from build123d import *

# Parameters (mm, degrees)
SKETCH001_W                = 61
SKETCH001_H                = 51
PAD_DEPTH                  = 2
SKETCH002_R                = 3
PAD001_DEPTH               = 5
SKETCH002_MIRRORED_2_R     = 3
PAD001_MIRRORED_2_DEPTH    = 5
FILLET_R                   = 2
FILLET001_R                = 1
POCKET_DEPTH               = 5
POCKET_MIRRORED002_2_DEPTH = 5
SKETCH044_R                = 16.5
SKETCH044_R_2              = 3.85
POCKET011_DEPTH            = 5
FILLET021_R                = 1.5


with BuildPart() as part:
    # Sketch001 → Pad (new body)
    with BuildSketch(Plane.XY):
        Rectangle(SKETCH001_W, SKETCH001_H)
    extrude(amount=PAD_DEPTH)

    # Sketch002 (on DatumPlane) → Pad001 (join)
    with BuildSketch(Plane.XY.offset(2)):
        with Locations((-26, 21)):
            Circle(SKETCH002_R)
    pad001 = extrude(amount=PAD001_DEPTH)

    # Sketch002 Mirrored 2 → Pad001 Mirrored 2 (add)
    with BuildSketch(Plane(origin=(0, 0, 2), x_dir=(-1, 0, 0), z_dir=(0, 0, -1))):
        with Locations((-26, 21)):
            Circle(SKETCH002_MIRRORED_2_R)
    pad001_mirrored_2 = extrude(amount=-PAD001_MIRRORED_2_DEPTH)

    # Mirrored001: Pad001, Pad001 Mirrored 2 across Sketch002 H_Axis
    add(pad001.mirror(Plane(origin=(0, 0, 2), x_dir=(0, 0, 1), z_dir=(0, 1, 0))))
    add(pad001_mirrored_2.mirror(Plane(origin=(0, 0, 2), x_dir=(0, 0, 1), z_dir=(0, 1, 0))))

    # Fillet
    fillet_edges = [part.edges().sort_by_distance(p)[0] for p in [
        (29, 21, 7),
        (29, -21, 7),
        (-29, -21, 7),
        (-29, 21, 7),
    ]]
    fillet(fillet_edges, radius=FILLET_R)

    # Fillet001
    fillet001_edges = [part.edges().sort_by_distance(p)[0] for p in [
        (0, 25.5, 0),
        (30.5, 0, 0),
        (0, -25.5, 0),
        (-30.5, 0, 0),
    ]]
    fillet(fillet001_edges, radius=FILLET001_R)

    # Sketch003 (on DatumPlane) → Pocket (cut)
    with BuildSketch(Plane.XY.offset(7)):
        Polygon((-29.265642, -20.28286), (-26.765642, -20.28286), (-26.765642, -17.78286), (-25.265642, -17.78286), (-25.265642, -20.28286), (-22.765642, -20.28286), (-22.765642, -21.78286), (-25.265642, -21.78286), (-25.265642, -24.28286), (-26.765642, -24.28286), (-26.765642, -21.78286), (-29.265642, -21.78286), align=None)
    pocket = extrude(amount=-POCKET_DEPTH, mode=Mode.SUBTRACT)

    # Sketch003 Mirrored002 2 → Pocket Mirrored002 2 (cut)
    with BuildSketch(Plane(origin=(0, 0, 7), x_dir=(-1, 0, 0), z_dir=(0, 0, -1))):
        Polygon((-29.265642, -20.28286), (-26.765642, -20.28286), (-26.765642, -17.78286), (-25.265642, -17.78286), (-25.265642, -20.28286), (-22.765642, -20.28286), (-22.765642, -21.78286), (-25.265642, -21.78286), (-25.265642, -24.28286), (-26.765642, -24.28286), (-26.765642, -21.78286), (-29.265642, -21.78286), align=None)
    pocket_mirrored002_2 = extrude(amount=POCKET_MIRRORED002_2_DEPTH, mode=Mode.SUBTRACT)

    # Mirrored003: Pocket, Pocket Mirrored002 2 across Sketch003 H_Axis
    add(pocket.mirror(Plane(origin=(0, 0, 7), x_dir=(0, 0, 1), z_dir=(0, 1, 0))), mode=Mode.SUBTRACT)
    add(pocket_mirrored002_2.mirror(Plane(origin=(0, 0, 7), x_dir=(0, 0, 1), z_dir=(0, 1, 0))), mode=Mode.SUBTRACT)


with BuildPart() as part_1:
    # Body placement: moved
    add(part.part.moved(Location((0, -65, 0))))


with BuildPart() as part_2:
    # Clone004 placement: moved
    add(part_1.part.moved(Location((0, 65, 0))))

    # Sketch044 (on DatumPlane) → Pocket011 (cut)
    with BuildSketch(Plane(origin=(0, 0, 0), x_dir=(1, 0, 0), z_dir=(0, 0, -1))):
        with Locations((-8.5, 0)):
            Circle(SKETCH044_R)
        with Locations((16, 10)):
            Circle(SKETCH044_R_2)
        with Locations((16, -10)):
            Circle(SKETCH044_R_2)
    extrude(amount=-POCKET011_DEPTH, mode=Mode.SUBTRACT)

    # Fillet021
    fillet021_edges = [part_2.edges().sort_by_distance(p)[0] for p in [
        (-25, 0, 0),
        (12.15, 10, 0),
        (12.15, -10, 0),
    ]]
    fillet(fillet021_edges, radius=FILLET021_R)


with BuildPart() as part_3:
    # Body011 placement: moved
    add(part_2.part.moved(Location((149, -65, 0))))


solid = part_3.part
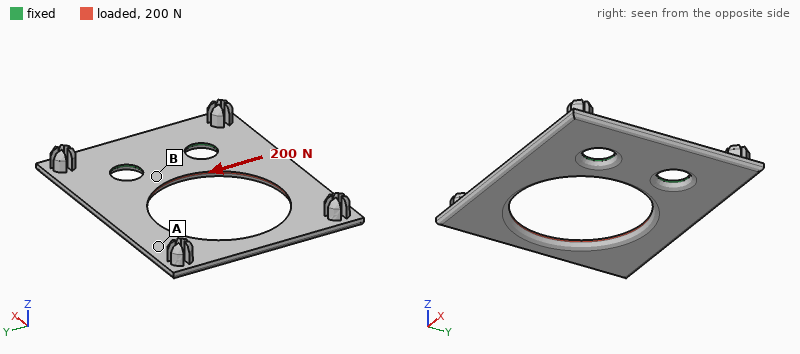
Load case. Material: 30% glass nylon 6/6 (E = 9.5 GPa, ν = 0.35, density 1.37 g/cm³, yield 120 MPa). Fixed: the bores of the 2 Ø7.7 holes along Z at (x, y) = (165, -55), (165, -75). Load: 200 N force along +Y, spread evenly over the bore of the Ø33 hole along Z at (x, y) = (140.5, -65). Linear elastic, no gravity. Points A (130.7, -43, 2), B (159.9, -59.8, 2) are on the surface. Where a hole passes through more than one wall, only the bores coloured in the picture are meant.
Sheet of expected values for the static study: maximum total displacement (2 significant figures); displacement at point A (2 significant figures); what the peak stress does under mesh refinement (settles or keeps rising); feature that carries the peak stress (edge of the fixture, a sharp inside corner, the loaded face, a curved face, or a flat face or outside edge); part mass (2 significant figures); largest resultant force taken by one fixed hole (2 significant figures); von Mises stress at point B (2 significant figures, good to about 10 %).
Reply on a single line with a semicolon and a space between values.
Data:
0.34 mm; 0.24 mm; keeps rising; edge of the fixture; 6.1 g; 170 N; 10 MPa
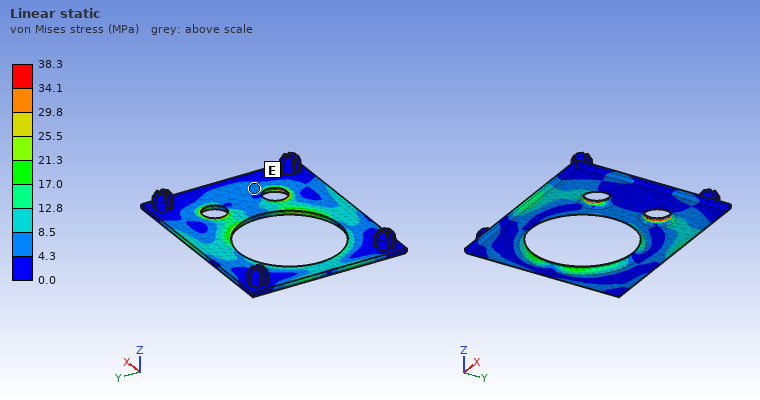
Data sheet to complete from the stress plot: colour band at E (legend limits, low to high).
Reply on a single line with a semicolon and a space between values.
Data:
4.3 to 8.5 MPa
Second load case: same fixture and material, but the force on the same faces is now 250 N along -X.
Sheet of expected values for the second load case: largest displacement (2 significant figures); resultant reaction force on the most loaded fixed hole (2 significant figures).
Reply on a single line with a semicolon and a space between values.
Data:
0.78 mm; 130 N
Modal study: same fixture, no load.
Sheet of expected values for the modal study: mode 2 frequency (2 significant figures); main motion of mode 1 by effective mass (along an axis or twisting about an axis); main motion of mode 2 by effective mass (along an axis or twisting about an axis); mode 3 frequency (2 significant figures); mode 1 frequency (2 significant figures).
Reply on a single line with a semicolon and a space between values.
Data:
610 Hz; along Z; twisting about X; 1700 Hz; 320 Hz
